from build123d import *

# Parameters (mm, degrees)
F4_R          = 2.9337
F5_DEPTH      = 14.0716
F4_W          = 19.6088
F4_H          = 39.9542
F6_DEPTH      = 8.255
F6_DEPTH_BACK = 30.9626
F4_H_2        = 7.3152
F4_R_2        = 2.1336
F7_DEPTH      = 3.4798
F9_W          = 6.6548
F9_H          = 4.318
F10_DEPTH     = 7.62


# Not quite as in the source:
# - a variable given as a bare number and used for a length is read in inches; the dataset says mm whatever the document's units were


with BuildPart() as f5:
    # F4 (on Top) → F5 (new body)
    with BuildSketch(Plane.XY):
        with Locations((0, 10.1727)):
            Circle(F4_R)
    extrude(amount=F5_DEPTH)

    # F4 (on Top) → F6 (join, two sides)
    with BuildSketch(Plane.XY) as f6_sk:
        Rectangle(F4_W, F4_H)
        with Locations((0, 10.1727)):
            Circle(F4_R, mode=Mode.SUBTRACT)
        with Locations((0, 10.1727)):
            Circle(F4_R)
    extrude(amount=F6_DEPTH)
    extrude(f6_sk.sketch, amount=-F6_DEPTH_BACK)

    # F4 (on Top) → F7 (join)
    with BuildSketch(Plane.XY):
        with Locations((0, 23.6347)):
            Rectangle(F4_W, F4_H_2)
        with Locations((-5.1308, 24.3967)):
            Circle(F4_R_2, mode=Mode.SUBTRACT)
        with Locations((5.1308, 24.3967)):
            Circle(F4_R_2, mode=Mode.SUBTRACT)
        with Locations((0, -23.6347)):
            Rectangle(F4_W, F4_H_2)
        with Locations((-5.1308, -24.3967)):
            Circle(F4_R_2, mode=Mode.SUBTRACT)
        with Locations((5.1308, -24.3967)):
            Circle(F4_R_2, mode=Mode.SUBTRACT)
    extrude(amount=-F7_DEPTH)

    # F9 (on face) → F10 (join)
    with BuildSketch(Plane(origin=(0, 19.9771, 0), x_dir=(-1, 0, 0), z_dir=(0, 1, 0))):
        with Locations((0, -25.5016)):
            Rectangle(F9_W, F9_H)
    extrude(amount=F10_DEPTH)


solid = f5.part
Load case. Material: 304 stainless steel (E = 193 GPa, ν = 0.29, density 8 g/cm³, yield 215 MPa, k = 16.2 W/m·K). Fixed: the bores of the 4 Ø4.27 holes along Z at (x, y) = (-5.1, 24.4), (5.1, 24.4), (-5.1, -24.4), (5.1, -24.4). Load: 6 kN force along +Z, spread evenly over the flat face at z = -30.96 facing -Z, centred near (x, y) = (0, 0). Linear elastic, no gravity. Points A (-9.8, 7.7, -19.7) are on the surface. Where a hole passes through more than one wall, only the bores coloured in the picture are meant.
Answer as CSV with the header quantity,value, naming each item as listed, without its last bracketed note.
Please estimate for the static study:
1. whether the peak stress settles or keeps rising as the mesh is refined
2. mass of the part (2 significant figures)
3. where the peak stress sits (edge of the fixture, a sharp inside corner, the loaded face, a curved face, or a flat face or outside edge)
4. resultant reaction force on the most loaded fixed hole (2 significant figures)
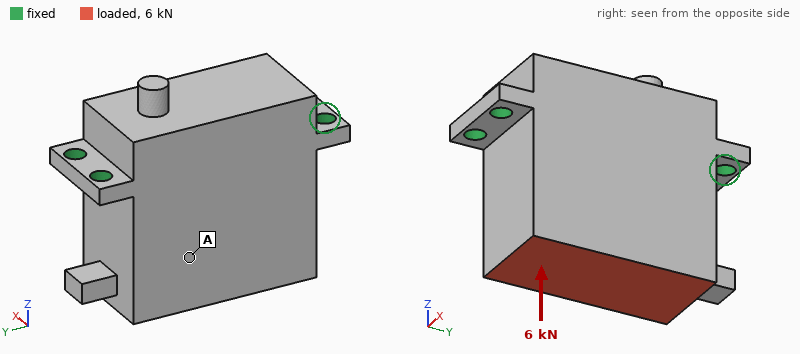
quantity,value
whether the peak stress settles or keeps rising as the mesh is refined,keeps rising
mass of the part,260 g
where the peak stress sits,edge of the fixture
resultant reaction force on the most loaded fixed hole,1.5 kN
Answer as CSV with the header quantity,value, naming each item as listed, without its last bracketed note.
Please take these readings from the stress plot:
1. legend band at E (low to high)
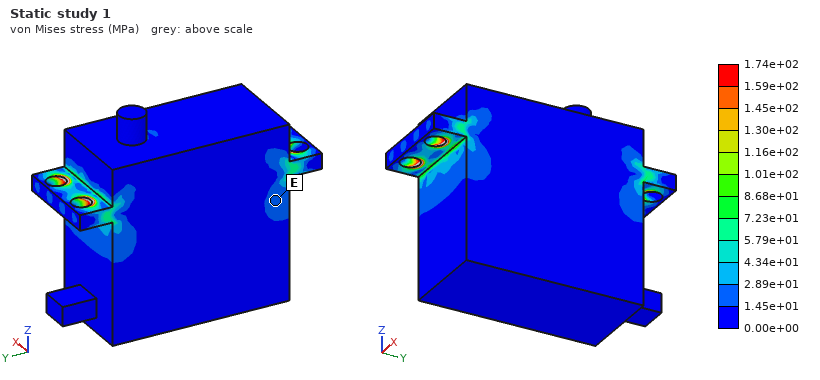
quantity,value
legend band at E,1.45e+01 to 2.89e+01 MPa
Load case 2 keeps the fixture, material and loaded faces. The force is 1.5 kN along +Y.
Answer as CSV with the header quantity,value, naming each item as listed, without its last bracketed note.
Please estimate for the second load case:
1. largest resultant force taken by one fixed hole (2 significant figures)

quantity,value
largest resultant force taken by one fixed hole,640 N
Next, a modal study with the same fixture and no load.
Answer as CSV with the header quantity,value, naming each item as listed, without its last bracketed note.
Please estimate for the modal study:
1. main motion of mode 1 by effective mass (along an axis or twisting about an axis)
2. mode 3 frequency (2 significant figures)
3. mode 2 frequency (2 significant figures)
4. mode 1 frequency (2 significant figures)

quantity,value
main motion of mode 1 by effective mass,along X
mode 3 frequency,11 kHz
mode 2 frequency,11 kHz
mode 1 frequency,4000 Hz
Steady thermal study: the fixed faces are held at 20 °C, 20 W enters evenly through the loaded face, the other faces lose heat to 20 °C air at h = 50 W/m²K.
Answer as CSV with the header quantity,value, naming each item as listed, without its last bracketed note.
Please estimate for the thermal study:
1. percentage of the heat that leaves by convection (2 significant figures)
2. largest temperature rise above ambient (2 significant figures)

quantity,value
percentage of the heat that leaves by convection,50 %
largest temperature rise above ambient,63 K
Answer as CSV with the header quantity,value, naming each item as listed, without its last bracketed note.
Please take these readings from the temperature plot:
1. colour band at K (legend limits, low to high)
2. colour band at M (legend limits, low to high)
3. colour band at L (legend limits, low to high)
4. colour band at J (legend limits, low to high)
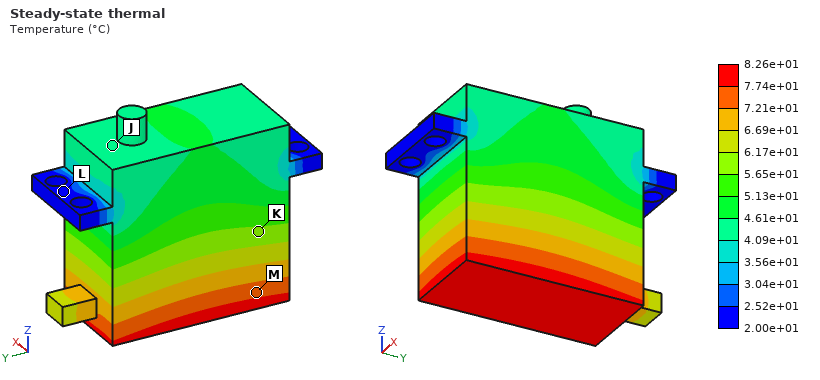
quantity,value
colour band at K,5.65e+01 to 6.17e+01 °C
colour band at M,7.21e+01 to 7.74e+01 °C
colour band at L,2.00e+01 to 2.52e+01 °C
colour band at J,4.09e+01 to 4.61e+01 °C
